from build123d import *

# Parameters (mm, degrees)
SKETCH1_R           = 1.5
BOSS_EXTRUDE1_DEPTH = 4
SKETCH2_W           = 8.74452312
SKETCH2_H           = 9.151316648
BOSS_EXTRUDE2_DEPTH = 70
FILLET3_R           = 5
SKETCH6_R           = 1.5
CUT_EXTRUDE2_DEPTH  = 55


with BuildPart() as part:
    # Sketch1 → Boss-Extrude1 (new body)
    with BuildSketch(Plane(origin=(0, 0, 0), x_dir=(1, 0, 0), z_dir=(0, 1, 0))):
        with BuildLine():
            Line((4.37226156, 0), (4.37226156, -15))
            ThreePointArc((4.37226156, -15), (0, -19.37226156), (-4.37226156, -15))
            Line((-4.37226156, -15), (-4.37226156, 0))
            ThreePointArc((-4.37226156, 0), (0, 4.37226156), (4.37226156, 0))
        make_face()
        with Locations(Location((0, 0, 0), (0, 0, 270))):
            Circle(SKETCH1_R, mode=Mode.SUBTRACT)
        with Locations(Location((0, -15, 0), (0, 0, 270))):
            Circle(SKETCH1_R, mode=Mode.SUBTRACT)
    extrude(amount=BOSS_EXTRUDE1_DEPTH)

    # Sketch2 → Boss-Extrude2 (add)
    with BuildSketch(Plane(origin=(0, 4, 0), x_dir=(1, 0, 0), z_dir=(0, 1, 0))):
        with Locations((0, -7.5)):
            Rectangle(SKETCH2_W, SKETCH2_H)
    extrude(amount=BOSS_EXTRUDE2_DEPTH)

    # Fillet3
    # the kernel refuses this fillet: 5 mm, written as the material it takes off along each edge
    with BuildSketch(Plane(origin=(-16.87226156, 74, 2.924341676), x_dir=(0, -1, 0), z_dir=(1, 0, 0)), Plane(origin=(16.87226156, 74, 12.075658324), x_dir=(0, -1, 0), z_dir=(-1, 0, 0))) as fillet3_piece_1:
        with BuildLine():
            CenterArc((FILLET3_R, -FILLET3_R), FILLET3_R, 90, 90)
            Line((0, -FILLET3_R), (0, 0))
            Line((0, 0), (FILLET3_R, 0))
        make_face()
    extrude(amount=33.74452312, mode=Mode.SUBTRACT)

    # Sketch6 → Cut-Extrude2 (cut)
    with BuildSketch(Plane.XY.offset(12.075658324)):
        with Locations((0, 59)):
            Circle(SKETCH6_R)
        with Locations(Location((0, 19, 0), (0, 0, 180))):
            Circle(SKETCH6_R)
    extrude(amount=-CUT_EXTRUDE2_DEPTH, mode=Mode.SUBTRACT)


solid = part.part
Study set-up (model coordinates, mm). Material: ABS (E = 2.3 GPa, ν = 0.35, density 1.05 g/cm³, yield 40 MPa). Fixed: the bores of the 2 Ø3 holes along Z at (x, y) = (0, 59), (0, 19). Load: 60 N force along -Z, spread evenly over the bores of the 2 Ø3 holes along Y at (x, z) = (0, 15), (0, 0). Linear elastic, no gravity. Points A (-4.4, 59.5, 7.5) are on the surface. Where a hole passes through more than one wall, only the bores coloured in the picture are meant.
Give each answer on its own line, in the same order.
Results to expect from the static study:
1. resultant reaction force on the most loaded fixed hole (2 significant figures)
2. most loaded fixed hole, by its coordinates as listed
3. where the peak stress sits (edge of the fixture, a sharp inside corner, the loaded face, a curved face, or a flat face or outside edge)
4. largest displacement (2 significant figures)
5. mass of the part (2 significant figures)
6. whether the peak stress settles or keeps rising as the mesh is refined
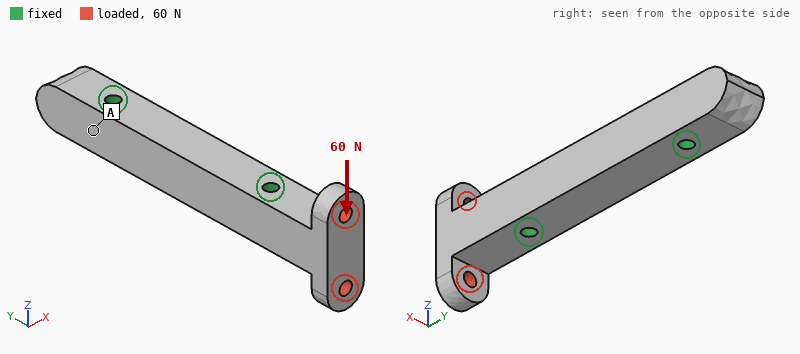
62 N
(0, 19)
edge of the fixture
0.14 mm
6.4 g
keeps rising
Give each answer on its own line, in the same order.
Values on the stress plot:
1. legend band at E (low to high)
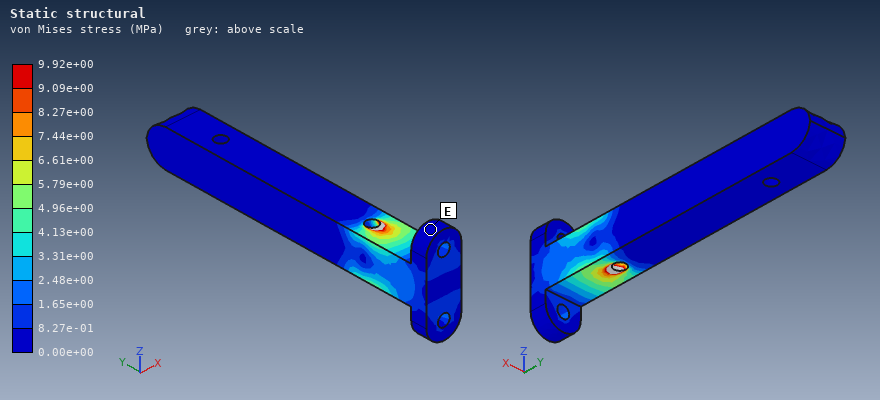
0.00e+00 to 8.27e-01 MPa
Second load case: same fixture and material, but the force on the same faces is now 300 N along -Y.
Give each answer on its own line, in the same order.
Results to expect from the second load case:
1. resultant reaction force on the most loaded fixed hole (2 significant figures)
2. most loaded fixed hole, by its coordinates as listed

290 N
(0, 19)
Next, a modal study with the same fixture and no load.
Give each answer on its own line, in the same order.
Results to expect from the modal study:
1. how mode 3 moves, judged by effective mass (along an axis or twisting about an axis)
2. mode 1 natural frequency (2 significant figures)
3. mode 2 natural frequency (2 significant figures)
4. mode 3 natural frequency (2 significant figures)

twisting about Y
3200 Hz
3800 Hz
5500 Hz
